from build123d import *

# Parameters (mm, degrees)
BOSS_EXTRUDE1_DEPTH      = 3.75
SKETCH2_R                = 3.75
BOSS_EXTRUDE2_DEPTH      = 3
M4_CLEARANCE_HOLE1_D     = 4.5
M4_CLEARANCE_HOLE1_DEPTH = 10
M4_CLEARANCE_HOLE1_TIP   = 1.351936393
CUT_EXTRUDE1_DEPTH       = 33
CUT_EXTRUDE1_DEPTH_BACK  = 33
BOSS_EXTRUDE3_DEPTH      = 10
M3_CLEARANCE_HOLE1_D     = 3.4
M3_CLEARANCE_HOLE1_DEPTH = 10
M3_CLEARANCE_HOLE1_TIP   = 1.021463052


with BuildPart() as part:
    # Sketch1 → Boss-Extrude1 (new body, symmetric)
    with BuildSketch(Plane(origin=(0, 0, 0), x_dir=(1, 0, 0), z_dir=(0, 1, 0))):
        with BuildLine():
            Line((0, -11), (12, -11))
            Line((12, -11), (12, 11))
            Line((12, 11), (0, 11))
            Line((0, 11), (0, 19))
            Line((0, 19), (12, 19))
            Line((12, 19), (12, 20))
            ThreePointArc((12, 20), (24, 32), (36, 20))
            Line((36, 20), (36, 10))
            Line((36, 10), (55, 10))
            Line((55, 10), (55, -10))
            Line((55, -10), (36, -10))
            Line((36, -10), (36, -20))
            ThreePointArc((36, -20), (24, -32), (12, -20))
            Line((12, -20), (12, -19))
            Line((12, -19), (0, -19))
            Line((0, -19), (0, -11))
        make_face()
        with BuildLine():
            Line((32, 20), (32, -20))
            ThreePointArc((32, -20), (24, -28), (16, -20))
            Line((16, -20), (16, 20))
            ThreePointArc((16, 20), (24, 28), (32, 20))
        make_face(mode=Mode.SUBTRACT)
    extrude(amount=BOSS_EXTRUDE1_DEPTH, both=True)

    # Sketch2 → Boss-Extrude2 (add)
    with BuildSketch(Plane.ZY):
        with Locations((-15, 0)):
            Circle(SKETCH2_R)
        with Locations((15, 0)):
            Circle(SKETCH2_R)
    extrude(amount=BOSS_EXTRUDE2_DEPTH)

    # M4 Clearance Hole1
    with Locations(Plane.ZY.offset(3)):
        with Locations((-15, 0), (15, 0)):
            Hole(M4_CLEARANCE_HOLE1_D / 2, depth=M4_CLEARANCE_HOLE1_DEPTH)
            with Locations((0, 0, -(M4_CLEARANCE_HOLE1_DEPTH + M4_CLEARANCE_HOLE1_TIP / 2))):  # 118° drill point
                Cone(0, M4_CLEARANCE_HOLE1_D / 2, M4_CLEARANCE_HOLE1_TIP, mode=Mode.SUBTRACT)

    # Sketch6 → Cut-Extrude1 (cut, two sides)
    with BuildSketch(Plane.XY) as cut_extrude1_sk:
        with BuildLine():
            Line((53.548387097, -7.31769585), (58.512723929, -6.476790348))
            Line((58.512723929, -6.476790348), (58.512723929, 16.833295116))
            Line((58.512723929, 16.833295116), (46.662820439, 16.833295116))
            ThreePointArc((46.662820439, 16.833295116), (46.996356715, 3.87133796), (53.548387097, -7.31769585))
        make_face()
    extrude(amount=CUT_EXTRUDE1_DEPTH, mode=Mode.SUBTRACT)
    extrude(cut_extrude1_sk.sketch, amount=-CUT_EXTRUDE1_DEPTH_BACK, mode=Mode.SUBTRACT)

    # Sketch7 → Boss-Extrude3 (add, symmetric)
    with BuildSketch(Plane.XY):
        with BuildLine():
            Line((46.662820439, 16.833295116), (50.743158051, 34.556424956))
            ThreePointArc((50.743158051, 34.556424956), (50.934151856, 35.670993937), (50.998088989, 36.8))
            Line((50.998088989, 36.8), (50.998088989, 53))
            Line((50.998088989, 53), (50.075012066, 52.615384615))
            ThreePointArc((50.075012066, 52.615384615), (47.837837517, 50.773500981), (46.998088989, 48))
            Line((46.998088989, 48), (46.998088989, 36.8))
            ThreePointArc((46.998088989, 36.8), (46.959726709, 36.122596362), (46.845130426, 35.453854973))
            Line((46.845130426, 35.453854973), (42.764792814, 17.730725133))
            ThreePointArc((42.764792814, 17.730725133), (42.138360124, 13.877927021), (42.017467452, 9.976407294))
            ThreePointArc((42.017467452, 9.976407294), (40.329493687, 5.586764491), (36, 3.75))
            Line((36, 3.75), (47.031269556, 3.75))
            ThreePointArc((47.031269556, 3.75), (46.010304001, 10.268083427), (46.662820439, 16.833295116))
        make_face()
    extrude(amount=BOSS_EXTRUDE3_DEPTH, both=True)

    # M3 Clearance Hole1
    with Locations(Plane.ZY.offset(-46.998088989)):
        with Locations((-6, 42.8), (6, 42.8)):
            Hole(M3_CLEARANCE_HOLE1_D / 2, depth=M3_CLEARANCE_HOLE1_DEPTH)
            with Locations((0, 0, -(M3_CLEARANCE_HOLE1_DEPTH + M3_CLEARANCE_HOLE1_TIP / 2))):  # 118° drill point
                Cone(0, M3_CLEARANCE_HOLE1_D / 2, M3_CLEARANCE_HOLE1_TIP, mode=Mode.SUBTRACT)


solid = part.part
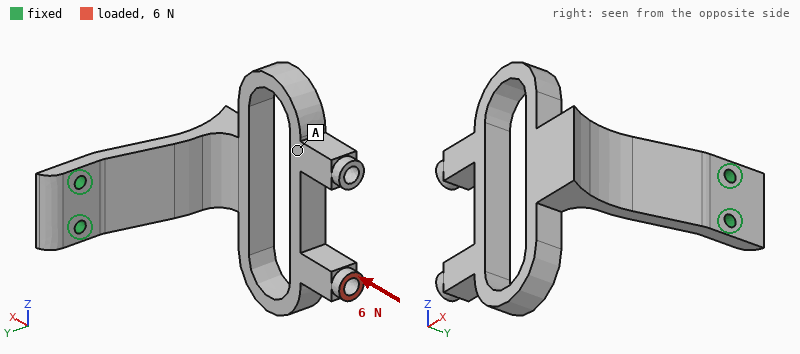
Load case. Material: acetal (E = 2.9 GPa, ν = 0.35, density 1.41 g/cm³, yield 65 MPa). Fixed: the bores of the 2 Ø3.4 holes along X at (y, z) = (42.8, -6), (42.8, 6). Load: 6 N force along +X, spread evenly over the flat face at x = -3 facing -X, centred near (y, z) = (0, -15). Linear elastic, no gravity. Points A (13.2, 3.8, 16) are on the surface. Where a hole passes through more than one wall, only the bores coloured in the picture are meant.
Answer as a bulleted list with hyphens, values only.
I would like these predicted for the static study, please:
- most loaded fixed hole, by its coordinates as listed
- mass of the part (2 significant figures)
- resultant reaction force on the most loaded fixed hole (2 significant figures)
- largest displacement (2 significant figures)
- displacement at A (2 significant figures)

- (42.8, -6)
- 16 g
- 9.2 N
- 1.2 mm
- 0.69 mm
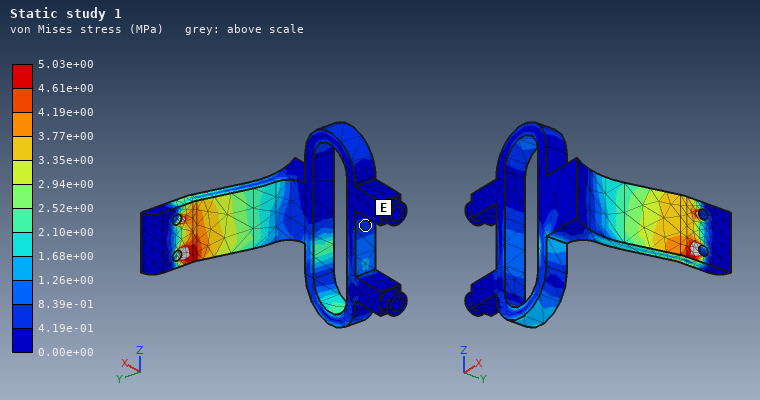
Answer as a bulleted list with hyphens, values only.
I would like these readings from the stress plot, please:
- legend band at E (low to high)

- 4.19e-01 to 8.39e-01 MPa
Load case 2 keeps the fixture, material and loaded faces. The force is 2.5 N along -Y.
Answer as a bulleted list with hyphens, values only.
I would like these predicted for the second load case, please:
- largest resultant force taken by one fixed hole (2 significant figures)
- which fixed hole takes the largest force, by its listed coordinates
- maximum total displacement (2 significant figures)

- 4.2 N
- (42.8, -6)
- 1.2 mm
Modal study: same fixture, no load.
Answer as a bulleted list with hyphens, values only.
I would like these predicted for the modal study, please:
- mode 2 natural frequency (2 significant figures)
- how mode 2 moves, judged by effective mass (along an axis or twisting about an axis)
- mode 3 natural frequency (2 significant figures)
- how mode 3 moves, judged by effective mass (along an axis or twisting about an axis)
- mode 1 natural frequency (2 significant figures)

- 190 Hz
- along Z
- 350 Hz
- along X
- 120 Hz
